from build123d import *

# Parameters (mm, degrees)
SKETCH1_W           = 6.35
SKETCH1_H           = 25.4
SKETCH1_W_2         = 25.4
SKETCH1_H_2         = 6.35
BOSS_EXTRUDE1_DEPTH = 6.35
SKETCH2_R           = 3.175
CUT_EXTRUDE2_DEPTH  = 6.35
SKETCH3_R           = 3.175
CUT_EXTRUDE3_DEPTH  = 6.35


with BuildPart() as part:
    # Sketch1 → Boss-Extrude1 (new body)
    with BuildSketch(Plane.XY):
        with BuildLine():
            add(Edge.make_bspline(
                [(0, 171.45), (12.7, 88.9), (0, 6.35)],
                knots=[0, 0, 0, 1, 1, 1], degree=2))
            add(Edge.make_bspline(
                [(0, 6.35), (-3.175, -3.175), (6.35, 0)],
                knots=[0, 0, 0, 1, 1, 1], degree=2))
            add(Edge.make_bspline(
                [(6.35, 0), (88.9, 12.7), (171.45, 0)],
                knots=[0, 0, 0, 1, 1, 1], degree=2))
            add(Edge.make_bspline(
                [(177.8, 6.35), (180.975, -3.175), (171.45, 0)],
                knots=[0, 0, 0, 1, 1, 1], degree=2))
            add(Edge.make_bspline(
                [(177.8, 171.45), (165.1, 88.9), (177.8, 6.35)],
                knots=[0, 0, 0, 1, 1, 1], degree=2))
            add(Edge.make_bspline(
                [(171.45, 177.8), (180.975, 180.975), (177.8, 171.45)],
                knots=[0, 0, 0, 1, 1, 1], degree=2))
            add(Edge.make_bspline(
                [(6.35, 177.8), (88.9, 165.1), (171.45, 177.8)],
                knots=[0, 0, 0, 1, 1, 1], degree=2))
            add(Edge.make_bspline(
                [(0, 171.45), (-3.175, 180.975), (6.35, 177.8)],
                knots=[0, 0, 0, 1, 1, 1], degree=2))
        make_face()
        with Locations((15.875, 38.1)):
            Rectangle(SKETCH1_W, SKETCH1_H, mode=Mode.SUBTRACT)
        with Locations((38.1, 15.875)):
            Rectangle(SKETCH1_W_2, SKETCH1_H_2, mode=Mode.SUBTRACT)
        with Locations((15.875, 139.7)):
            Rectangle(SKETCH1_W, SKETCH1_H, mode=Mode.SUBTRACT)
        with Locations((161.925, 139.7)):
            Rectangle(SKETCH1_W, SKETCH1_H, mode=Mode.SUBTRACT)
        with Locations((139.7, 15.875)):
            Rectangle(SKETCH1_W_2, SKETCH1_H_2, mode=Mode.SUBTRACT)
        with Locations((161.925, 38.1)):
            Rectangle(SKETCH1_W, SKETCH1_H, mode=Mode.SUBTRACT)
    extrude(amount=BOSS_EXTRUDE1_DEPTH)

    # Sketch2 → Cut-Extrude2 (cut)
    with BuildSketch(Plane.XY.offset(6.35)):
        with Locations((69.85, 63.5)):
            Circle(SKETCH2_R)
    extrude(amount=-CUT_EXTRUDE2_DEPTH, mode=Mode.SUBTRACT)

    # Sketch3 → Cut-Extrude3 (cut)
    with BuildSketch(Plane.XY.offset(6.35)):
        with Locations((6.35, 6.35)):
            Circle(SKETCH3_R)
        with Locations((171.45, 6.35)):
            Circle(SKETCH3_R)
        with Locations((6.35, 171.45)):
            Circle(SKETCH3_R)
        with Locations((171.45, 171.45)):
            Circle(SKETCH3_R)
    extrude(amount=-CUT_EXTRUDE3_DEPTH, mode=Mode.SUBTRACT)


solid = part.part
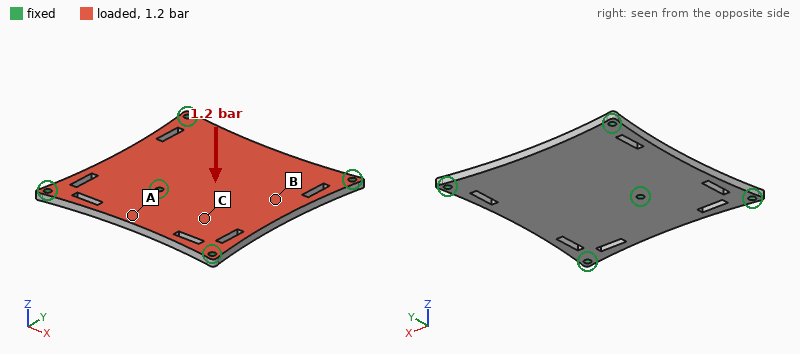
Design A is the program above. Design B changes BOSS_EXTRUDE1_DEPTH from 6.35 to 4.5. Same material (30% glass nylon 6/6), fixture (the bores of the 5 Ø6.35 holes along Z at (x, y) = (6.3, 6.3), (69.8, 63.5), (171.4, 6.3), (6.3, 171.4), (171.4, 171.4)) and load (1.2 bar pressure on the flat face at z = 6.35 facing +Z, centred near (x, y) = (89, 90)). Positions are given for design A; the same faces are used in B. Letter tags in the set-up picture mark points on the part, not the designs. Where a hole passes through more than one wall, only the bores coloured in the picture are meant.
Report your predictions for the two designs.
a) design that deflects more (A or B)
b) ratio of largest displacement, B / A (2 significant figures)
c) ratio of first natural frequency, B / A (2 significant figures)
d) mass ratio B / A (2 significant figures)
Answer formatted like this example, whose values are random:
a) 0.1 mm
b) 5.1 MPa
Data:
a) B
b) 2.7
c) 0.73
d) 0.71
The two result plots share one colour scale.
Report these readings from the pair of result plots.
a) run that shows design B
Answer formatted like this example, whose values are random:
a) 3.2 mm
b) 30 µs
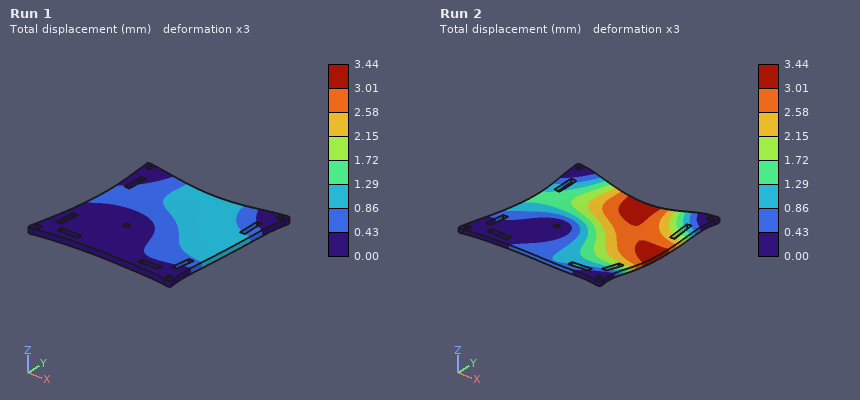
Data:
a) Run 2
